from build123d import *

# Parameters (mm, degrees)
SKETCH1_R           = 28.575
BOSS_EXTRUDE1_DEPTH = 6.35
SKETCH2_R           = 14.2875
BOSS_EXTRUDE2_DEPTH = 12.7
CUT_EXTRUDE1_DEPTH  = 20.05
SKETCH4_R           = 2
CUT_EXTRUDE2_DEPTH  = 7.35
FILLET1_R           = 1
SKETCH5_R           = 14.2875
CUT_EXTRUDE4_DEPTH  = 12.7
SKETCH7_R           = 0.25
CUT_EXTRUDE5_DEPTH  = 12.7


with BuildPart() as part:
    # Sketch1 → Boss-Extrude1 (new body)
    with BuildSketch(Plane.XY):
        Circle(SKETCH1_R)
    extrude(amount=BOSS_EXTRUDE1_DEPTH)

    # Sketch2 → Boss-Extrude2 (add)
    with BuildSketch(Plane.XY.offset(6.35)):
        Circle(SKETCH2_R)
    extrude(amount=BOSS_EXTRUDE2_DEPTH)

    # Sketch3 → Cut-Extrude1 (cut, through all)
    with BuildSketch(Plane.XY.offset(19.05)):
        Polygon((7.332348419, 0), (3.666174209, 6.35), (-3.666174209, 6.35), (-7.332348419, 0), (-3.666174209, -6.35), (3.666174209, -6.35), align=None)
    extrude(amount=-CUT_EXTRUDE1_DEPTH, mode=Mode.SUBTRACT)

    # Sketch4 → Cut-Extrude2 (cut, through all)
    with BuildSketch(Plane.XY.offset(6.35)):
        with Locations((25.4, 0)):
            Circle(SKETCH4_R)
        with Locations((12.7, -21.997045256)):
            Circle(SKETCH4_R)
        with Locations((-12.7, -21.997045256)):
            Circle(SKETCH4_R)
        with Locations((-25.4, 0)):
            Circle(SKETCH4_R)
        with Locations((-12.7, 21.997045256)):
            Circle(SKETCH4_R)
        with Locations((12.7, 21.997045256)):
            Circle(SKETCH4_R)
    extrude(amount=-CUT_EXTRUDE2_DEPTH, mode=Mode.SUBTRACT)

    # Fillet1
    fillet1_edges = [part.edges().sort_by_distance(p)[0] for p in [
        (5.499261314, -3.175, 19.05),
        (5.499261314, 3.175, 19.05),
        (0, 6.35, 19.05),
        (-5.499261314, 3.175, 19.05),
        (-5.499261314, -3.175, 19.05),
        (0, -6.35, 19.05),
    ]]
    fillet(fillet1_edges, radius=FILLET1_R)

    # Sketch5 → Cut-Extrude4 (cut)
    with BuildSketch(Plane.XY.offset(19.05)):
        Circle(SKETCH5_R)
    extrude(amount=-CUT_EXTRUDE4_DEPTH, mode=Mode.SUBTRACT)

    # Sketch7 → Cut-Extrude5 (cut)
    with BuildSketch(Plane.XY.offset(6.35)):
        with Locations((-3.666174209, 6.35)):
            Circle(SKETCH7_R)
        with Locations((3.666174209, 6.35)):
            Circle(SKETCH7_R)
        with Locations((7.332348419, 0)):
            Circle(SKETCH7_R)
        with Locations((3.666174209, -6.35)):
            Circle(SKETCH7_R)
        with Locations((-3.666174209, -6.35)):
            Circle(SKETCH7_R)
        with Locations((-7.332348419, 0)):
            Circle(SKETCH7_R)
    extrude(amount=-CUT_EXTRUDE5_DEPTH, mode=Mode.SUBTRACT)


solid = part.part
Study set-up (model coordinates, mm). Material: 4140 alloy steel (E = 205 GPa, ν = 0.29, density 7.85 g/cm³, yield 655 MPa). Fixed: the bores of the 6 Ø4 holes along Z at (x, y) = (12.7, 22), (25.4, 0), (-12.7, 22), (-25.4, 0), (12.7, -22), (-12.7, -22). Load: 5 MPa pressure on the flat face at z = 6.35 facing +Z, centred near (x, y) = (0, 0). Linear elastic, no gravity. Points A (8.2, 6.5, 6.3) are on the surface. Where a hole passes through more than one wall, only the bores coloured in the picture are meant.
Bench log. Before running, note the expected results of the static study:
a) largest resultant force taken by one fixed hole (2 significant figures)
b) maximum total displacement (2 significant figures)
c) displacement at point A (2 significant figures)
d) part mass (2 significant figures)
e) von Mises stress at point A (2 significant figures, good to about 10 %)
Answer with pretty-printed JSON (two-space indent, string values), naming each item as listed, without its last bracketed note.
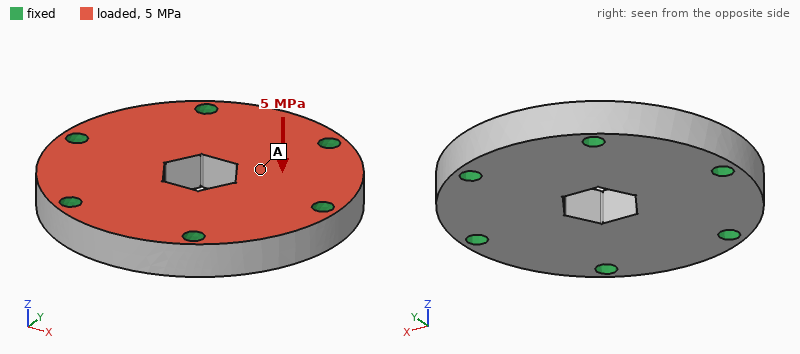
{
  "largest resultant force taken by one fixed hole": "2.0 kN",
  "maximum total displacement": "11 µm",
  "displacement at point A": "8.6 µm",
  "part mass": "120 g",
  "von Mises stress at point A": "31 MPa"
}
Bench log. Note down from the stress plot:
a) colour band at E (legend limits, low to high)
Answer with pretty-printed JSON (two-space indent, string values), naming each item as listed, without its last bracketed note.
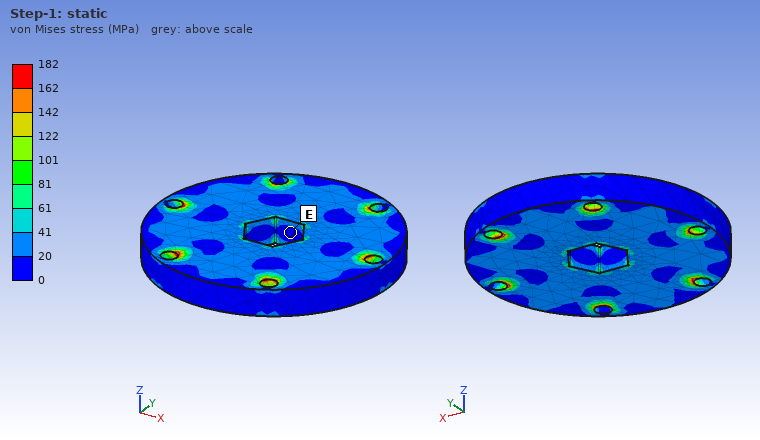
{
  "colour band at E": "0 to 20 MPa"
}
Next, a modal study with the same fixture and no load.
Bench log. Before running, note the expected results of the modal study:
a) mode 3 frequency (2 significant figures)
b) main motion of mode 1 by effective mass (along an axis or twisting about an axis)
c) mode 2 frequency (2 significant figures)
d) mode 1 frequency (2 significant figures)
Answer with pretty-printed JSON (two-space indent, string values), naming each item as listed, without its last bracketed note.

{
  "mode 3 frequency": "32 kHz",
  "main motion of mode 1 by effective mass": "along Z",
  "mode 2 frequency": "32 kHz",
  "mode 1 frequency": "19 kHz"
}
